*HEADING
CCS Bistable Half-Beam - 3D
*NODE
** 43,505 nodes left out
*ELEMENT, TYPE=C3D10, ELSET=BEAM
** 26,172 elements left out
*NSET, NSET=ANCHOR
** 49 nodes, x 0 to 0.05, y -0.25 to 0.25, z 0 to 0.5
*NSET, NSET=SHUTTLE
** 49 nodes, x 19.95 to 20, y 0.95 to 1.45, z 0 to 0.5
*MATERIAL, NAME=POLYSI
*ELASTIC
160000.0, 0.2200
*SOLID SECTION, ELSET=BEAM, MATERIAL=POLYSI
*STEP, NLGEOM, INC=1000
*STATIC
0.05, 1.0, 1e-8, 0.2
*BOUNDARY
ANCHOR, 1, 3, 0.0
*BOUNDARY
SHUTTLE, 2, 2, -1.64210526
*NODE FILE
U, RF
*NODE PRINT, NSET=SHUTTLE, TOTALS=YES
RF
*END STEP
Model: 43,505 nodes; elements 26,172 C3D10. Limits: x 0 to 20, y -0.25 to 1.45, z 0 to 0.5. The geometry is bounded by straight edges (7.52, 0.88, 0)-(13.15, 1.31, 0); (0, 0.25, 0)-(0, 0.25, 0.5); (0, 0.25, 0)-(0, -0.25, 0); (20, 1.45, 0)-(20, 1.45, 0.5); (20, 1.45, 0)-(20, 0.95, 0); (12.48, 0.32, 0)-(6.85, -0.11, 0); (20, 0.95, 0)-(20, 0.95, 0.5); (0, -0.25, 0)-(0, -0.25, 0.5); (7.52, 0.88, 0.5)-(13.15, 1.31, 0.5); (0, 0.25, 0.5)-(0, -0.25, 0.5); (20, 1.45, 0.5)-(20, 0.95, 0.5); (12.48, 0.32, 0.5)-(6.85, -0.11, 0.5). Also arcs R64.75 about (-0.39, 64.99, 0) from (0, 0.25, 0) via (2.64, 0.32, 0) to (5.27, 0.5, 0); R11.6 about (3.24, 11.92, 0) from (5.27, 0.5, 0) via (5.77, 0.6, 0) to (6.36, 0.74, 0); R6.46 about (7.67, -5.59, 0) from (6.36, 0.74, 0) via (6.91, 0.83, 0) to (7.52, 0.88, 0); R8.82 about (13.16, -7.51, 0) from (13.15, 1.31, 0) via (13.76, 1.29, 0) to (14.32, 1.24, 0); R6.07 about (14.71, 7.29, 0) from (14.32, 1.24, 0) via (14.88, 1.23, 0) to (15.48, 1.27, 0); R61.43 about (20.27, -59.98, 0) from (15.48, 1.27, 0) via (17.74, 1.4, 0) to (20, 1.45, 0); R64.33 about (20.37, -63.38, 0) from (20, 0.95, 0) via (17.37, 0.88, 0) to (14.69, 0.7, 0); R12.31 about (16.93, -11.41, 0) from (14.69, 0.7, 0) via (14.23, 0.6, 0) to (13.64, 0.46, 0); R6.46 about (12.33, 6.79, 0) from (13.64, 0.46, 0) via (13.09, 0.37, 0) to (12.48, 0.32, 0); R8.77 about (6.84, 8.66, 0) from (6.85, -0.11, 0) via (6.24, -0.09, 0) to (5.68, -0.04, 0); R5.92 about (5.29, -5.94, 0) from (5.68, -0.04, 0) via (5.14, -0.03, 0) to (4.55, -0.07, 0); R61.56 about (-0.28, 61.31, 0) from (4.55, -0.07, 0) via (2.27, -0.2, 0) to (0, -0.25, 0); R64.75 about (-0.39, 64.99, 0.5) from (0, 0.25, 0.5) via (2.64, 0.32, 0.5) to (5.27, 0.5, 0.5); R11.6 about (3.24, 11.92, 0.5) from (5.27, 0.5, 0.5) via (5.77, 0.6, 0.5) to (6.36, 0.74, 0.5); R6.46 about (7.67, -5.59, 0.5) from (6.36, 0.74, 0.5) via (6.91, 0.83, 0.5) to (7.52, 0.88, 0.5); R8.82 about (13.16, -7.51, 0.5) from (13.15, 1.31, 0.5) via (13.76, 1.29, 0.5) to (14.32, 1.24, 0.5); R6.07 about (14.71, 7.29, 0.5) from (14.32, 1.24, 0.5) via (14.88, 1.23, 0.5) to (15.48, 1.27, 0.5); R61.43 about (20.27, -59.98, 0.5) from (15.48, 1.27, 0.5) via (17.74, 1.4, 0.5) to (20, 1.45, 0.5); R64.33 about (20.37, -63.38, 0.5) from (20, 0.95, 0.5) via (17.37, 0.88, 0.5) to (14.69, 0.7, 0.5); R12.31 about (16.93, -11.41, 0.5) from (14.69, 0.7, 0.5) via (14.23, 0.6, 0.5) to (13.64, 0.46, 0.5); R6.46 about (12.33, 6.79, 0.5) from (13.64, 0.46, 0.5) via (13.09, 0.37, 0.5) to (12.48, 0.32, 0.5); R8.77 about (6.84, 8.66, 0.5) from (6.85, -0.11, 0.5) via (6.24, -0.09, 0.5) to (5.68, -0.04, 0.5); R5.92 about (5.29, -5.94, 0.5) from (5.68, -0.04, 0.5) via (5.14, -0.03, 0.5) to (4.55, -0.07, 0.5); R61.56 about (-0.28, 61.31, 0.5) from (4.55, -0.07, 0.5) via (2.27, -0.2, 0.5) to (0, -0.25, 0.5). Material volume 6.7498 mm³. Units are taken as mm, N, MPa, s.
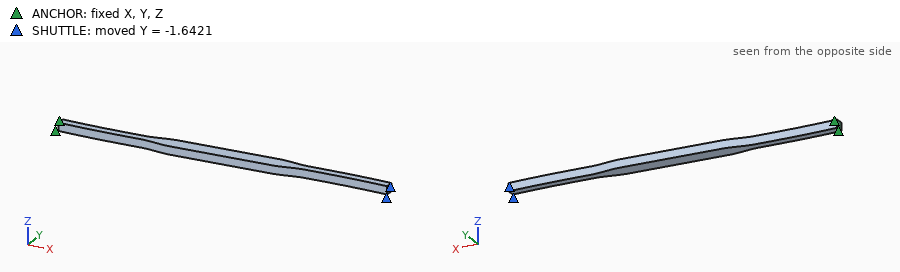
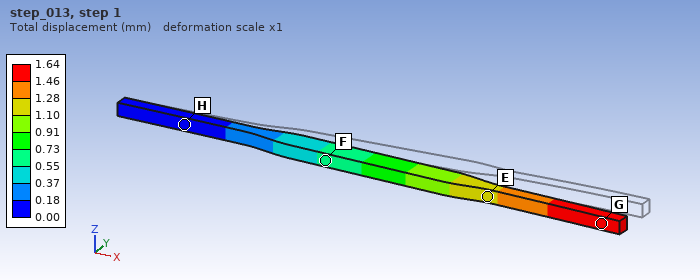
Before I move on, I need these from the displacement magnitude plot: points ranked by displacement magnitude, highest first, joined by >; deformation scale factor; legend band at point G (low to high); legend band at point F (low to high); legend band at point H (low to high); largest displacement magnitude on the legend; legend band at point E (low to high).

G > E > F > H
1
1.46 to 1.64 mm
0.55 to 0.73 mm
0.00 to 0.18 mm
1.64 mm
1.10 to 1.28 mm
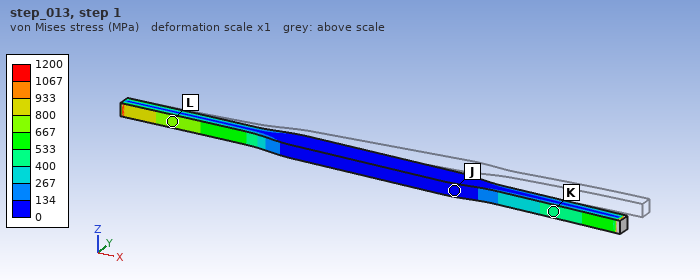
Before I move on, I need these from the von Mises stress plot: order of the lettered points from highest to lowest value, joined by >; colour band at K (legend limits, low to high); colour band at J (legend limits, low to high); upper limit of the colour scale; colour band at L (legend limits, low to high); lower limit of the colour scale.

L > K > J
400 to 533 MPa
0 to 134 MPa
1200 MPa
667 to 800 MPa
0 MPa
